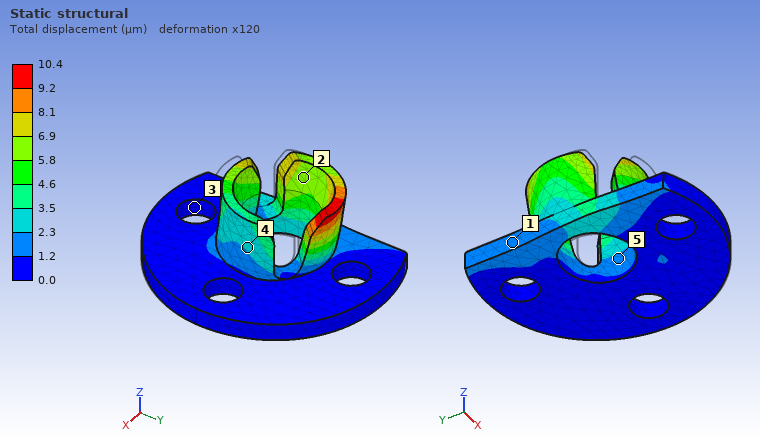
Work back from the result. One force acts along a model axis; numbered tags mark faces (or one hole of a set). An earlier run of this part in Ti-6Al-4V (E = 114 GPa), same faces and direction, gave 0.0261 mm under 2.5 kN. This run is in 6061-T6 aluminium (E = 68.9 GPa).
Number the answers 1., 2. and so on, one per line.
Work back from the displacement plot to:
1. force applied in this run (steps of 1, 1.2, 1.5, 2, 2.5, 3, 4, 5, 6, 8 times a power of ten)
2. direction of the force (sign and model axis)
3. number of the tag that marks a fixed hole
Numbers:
1. 600 N
2. +Y
3. 3
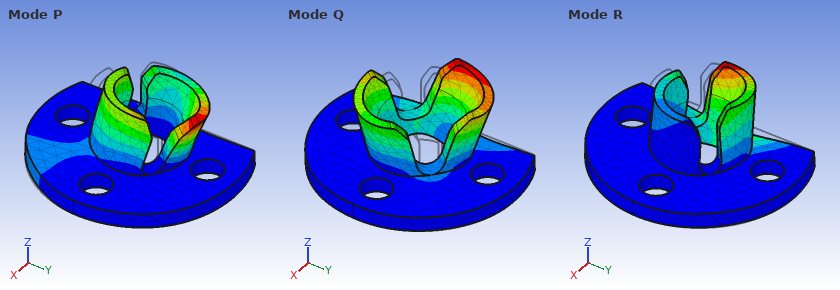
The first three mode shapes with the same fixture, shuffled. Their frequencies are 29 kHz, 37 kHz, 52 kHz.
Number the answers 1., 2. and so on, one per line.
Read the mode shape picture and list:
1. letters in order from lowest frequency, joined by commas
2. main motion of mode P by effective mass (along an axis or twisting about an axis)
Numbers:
1. R, Q, P
2. along Y
